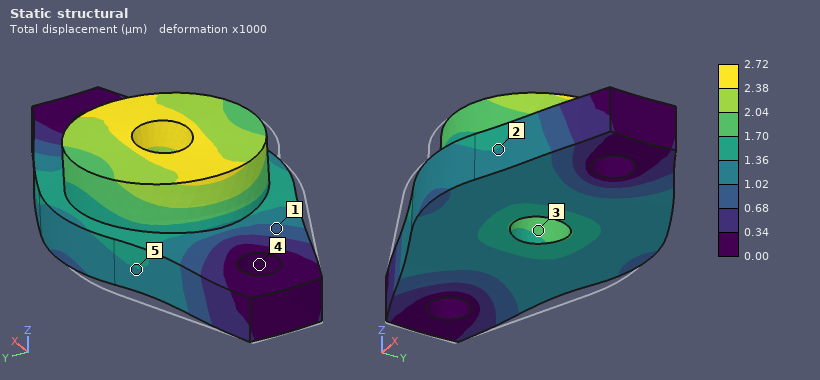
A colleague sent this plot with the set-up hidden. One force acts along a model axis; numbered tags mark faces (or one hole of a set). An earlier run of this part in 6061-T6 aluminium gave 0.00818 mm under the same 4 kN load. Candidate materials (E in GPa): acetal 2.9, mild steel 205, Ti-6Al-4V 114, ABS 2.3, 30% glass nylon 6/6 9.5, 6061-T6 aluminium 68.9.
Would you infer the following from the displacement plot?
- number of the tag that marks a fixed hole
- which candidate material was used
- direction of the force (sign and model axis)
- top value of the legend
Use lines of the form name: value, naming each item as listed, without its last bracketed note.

number of the tag that marks a fixed hole: 4
which candidate material was used: mild steel
direction of the force: +X
top value of the legend: 2.72 µm
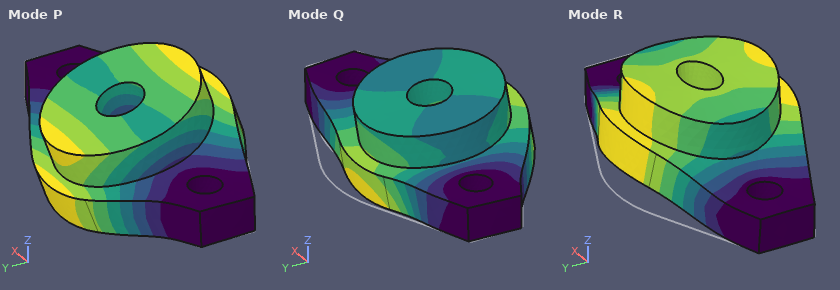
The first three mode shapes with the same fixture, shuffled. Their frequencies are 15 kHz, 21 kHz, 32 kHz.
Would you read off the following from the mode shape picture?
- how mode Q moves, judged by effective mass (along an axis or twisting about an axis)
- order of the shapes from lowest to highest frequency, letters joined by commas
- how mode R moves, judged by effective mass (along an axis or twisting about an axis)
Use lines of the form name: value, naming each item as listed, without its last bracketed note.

how mode Q moves, judged by effective mass: along Y
order of the shapes from lowest to highest frequency, letters joined by commas: P, R, Q
how mode R moves, judged by effective mass: along Z
